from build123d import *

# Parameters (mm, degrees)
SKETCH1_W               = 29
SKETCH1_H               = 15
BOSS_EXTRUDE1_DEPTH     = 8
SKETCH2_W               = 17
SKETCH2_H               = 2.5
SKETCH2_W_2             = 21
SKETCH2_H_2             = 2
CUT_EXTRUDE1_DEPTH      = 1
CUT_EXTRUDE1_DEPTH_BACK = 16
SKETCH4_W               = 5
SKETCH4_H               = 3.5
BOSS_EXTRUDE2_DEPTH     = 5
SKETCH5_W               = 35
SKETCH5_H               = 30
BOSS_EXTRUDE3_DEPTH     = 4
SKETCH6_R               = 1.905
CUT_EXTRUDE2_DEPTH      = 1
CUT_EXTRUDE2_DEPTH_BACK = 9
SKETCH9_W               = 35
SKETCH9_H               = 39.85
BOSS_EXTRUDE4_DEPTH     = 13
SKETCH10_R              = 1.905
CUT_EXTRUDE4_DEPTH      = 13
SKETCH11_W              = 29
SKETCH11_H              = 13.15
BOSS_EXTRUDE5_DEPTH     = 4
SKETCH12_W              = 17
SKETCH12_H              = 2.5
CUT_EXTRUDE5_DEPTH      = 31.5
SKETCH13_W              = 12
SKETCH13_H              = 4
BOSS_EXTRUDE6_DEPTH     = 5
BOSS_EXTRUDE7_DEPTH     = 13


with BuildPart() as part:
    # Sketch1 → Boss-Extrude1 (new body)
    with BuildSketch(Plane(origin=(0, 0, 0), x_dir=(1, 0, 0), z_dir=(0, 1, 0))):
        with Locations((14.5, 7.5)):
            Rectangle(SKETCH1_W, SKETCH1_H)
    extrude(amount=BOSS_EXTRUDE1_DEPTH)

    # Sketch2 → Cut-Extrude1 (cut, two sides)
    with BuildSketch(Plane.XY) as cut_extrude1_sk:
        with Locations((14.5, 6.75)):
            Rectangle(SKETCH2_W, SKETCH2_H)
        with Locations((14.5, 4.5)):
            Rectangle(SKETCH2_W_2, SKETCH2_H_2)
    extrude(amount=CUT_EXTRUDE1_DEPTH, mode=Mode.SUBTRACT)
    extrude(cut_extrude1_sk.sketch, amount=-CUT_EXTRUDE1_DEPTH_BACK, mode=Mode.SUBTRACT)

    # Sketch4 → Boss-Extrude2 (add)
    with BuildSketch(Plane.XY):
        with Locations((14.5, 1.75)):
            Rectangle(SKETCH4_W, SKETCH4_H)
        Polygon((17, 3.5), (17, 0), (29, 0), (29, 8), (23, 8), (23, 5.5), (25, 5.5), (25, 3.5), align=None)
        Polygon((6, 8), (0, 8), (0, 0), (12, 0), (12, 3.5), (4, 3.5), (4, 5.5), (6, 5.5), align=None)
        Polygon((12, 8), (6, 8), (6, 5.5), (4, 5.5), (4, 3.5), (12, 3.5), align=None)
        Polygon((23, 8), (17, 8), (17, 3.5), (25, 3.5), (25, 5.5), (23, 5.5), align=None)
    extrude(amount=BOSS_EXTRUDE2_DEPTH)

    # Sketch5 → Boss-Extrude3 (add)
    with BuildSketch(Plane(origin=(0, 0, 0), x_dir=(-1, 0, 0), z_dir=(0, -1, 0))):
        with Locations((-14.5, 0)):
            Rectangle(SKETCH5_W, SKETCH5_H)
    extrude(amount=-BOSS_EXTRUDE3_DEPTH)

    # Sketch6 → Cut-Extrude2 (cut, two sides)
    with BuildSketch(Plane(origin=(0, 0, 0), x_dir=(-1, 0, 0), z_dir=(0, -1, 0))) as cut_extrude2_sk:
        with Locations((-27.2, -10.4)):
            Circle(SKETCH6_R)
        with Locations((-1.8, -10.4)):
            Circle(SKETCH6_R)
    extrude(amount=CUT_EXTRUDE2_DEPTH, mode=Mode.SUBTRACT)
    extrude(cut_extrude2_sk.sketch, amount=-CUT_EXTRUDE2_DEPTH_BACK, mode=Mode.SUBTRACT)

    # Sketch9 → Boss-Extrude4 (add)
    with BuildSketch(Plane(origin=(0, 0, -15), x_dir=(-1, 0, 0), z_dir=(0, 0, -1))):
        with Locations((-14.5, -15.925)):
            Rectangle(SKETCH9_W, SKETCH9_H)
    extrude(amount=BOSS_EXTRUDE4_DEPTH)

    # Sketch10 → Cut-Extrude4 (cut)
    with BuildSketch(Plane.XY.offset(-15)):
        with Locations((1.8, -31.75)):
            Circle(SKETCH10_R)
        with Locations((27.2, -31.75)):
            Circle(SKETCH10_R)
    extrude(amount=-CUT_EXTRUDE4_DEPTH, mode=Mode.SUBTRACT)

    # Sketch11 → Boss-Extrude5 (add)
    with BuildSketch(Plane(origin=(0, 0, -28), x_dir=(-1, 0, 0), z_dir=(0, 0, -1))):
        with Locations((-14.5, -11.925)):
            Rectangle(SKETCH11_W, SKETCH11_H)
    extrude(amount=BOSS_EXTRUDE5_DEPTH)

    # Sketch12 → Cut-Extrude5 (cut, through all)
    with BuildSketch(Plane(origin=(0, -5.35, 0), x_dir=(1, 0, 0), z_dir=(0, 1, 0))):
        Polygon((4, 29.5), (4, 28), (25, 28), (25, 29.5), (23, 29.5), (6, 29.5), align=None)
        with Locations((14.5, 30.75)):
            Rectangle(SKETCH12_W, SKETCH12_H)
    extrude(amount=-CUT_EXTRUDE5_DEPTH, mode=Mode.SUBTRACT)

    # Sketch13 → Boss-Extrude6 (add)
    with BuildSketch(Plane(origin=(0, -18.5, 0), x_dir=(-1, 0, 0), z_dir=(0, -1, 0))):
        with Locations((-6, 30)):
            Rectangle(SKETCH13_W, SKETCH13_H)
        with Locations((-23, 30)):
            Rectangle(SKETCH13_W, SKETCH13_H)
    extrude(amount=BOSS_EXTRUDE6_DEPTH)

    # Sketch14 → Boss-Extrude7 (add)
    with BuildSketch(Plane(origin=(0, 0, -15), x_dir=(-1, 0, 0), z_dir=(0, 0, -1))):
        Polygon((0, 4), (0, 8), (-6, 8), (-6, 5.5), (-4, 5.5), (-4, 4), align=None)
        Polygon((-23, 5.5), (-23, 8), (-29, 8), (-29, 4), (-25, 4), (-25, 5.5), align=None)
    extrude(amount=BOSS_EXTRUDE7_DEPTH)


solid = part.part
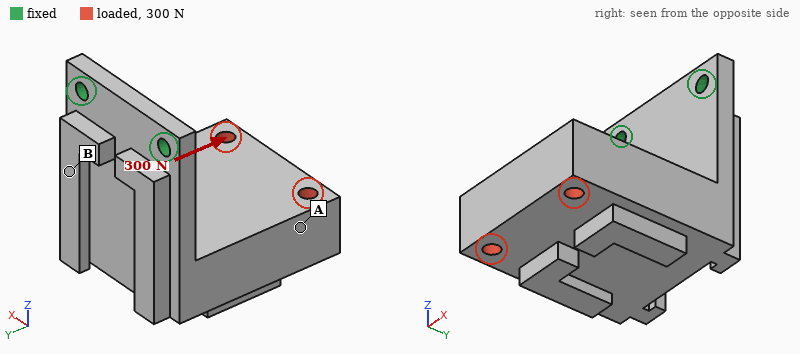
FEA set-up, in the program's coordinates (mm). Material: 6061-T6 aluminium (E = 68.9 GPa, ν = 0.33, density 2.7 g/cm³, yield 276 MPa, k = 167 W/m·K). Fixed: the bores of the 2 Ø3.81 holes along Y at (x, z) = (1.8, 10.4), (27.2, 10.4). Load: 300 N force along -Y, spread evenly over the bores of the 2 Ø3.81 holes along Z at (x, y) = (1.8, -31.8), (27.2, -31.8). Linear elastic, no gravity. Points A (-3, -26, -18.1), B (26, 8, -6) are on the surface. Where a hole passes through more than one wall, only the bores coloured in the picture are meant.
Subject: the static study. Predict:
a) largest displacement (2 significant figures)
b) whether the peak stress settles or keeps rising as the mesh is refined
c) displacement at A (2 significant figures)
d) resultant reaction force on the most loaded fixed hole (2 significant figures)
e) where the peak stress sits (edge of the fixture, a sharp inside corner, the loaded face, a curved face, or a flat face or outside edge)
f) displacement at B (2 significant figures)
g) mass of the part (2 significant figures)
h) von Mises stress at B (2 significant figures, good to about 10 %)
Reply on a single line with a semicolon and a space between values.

0.35 mm; keeps rising; 0.25 mm; 150 N; edge of the fixture; 0.082 mm; 67 g; 31 MPa
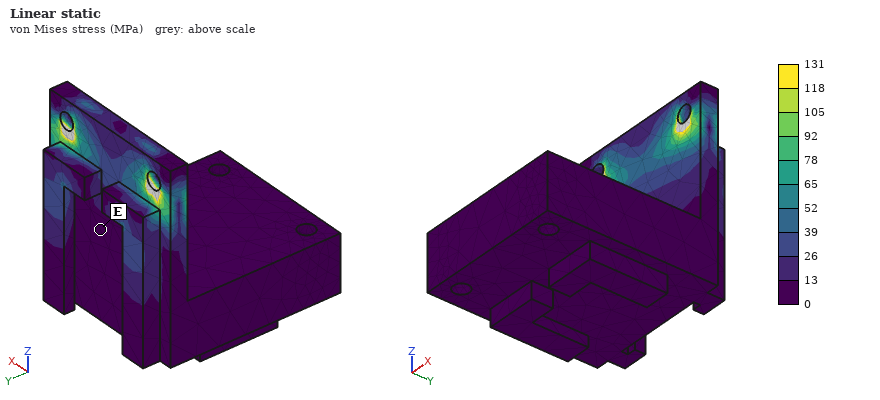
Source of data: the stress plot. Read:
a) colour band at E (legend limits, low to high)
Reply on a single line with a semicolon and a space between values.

0 to 13 MPa
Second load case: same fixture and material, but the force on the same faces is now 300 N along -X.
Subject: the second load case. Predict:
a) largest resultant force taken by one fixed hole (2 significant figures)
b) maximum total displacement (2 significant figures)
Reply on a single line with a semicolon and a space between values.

530 N; 0.17 mm
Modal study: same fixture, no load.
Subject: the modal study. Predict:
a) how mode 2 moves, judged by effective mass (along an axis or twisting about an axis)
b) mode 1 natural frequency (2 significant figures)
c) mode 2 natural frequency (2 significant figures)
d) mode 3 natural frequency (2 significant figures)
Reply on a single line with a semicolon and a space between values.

along X; 670 Hz; 1500 Hz; 3200 Hz
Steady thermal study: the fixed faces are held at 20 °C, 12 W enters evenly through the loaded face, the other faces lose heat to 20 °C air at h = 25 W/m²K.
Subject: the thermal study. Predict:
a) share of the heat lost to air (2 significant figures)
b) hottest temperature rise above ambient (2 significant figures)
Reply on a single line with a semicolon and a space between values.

18 %; 16 K
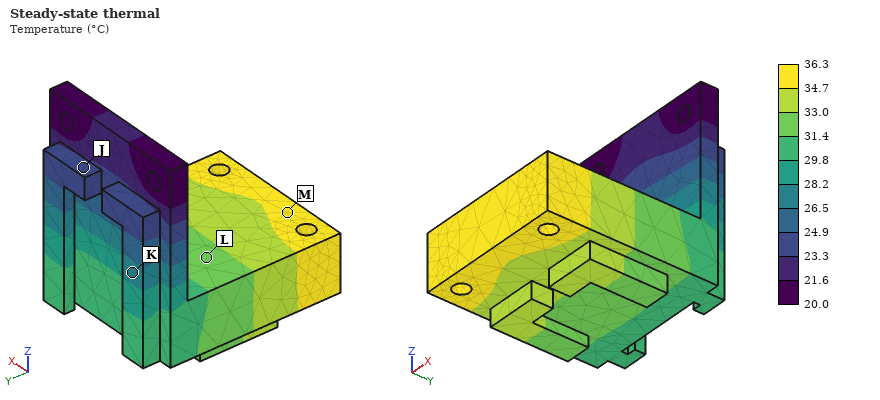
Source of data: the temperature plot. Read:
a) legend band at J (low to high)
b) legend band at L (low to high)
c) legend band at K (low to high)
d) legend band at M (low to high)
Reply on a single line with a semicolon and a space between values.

23.3 to 24.9 °C; 31.4 to 33.0 °C; 26.5 to 28.2 °C; 34.7 to 36.3 °C
